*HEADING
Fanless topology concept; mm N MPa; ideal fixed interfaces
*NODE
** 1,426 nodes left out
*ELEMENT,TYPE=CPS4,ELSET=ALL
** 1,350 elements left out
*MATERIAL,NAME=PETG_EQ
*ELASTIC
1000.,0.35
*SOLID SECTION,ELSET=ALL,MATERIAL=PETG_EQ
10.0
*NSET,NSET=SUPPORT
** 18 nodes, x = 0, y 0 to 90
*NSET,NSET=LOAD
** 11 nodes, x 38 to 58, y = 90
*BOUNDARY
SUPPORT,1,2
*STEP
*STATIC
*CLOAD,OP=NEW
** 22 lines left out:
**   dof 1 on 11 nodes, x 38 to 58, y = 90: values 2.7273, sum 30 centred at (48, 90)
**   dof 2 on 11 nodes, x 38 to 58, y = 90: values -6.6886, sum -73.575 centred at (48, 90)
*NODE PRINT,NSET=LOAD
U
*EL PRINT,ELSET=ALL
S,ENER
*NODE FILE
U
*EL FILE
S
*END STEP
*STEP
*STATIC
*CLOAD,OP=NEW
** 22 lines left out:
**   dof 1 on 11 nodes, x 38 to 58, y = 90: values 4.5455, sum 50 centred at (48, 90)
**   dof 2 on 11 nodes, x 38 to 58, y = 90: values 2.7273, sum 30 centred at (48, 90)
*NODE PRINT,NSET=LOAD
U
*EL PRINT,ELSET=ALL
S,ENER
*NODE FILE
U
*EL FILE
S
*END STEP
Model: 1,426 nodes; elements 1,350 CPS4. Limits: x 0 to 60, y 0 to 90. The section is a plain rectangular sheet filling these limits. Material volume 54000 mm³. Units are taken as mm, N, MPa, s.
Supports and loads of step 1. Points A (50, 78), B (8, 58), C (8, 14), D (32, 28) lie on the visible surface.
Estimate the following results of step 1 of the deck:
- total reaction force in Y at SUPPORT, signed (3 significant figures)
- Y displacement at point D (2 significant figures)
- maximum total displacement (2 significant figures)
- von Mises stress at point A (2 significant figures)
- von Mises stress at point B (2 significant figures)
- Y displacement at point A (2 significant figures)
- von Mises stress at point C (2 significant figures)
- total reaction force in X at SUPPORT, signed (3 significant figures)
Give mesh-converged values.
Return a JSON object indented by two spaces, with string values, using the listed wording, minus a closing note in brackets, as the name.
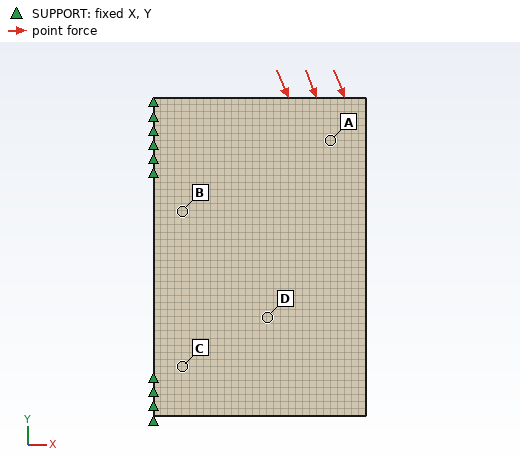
{
  "total reaction force in Y at SUPPORT, signed": "73.6 N",
  "Y displacement at point D": "-0.013 mm",
  "maximum total displacement": "0.048 mm",
  "von Mises stress at point A": "0.35 MPa",
  "von Mises stress at point B": "0.15 MPa",
  "Y displacement at point A": "-0.030 mm",
  "von Mises stress at point C": "0.30 MPa",
  "total reaction force in X at SUPPORT, signed": "-30.0 N"
}
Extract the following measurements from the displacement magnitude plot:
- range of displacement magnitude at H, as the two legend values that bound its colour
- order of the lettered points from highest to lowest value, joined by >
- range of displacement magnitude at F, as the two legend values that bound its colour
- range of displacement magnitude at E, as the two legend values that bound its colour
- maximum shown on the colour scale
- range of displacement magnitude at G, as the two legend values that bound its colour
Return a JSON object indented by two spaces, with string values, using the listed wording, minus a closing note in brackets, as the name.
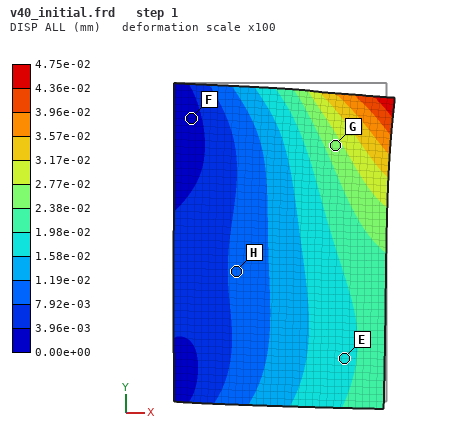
{
  "range of displacement magnitude at H, as the two legend values that bound its colour": "7.92e-03 to 1.19e-02 mm",
  "order of the lettered points from highest to lowest value, joined by >": "G > E > H > F",
  "range of displacement magnitude at F, as the two legend values that bound its colour": "0.00e+00 to 3.96e-03 mm",
  "range of displacement magnitude at E, as the two legend values that bound its colour": "1.58e-02 to 1.98e-02 mm",
  "maximum shown on the colour scale": "4.75e-02 mm",
  "range of displacement magnitude at G, as the two legend values that bound its colour": "2.38e-02 to 2.77e-02 mm"
}
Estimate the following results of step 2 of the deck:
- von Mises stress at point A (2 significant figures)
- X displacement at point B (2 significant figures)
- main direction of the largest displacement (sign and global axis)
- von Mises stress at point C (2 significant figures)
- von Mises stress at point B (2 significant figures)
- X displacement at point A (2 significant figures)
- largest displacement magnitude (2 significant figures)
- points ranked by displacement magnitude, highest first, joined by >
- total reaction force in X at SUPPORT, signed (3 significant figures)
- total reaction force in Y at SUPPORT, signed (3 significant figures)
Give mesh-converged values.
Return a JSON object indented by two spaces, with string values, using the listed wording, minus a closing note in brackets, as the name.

{
  "von Mises stress at point A": "0.095 MPa",
  "X displacement at point B": "0.0034 mm",
  "main direction of the largest displacement": "+X",
  "von Mises stress at point C": "0.096 MPa",
  "von Mises stress at point B": "0.059 MPa",
  "X displacement at point A": "0.0072 mm",
  "largest displacement magnitude": "0.017 mm",
  "points ranked by displacement magnitude, highest first, joined by >": "A > B > D > C",
  "total reaction force in X at SUPPORT, signed": "-50.0 N",
  "total reaction force in Y at SUPPORT, signed": "-30.0 N"
}
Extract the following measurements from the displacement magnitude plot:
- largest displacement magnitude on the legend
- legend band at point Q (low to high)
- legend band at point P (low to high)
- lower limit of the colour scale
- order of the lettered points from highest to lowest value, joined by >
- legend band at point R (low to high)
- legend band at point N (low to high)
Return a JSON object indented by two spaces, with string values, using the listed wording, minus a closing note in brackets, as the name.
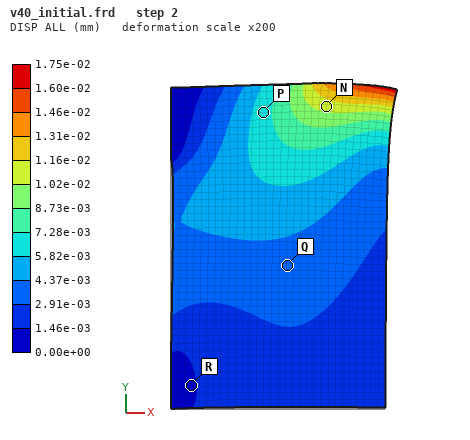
{
  "largest displacement magnitude on the legend": "1.75e-02 mm",
  "legend band at point Q": "2.91e-03 to 4.37e-03 mm",
  "legend band at point P": "5.82e-03 to 7.28e-03 mm",
  "lower limit of the colour scale": "0.00e+00 mm",
  "order of the lettered points from highest to lowest value, joined by >": "N > P > Q > R",
  "legend band at point R": "0.00e+00 to 1.46e-03 mm",
  "legend band at point N": "1.02e-02 to 1.16e-02 mm"
}
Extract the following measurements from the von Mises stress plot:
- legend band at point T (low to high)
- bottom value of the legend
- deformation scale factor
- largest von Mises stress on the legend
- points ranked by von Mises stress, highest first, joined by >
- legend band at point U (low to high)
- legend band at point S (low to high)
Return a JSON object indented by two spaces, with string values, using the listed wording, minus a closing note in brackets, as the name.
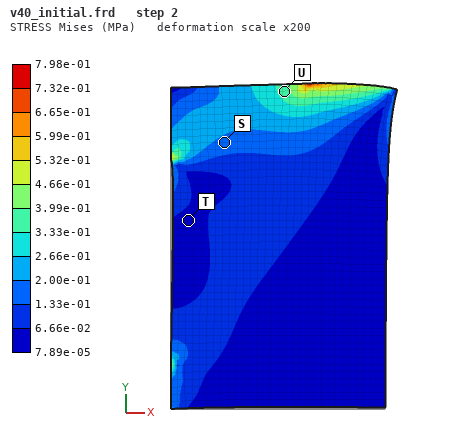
{
  "legend band at point T": "7.89e-05 to 6.66e-02 MPa",
  "bottom value of the legend": "7.89e-05 MPa",
  "deformation scale factor": "200",
  "largest von Mises stress on the legend": "7.98e-01 MPa",
  "points ranked by von Mises stress, highest first, joined by >": "U > S > T",
  "legend band at point U": "3.33e-01 to 3.99e-01 MPa",
  "legend band at point S": "1.33e-01 to 2.00e-01 MPa"
}
